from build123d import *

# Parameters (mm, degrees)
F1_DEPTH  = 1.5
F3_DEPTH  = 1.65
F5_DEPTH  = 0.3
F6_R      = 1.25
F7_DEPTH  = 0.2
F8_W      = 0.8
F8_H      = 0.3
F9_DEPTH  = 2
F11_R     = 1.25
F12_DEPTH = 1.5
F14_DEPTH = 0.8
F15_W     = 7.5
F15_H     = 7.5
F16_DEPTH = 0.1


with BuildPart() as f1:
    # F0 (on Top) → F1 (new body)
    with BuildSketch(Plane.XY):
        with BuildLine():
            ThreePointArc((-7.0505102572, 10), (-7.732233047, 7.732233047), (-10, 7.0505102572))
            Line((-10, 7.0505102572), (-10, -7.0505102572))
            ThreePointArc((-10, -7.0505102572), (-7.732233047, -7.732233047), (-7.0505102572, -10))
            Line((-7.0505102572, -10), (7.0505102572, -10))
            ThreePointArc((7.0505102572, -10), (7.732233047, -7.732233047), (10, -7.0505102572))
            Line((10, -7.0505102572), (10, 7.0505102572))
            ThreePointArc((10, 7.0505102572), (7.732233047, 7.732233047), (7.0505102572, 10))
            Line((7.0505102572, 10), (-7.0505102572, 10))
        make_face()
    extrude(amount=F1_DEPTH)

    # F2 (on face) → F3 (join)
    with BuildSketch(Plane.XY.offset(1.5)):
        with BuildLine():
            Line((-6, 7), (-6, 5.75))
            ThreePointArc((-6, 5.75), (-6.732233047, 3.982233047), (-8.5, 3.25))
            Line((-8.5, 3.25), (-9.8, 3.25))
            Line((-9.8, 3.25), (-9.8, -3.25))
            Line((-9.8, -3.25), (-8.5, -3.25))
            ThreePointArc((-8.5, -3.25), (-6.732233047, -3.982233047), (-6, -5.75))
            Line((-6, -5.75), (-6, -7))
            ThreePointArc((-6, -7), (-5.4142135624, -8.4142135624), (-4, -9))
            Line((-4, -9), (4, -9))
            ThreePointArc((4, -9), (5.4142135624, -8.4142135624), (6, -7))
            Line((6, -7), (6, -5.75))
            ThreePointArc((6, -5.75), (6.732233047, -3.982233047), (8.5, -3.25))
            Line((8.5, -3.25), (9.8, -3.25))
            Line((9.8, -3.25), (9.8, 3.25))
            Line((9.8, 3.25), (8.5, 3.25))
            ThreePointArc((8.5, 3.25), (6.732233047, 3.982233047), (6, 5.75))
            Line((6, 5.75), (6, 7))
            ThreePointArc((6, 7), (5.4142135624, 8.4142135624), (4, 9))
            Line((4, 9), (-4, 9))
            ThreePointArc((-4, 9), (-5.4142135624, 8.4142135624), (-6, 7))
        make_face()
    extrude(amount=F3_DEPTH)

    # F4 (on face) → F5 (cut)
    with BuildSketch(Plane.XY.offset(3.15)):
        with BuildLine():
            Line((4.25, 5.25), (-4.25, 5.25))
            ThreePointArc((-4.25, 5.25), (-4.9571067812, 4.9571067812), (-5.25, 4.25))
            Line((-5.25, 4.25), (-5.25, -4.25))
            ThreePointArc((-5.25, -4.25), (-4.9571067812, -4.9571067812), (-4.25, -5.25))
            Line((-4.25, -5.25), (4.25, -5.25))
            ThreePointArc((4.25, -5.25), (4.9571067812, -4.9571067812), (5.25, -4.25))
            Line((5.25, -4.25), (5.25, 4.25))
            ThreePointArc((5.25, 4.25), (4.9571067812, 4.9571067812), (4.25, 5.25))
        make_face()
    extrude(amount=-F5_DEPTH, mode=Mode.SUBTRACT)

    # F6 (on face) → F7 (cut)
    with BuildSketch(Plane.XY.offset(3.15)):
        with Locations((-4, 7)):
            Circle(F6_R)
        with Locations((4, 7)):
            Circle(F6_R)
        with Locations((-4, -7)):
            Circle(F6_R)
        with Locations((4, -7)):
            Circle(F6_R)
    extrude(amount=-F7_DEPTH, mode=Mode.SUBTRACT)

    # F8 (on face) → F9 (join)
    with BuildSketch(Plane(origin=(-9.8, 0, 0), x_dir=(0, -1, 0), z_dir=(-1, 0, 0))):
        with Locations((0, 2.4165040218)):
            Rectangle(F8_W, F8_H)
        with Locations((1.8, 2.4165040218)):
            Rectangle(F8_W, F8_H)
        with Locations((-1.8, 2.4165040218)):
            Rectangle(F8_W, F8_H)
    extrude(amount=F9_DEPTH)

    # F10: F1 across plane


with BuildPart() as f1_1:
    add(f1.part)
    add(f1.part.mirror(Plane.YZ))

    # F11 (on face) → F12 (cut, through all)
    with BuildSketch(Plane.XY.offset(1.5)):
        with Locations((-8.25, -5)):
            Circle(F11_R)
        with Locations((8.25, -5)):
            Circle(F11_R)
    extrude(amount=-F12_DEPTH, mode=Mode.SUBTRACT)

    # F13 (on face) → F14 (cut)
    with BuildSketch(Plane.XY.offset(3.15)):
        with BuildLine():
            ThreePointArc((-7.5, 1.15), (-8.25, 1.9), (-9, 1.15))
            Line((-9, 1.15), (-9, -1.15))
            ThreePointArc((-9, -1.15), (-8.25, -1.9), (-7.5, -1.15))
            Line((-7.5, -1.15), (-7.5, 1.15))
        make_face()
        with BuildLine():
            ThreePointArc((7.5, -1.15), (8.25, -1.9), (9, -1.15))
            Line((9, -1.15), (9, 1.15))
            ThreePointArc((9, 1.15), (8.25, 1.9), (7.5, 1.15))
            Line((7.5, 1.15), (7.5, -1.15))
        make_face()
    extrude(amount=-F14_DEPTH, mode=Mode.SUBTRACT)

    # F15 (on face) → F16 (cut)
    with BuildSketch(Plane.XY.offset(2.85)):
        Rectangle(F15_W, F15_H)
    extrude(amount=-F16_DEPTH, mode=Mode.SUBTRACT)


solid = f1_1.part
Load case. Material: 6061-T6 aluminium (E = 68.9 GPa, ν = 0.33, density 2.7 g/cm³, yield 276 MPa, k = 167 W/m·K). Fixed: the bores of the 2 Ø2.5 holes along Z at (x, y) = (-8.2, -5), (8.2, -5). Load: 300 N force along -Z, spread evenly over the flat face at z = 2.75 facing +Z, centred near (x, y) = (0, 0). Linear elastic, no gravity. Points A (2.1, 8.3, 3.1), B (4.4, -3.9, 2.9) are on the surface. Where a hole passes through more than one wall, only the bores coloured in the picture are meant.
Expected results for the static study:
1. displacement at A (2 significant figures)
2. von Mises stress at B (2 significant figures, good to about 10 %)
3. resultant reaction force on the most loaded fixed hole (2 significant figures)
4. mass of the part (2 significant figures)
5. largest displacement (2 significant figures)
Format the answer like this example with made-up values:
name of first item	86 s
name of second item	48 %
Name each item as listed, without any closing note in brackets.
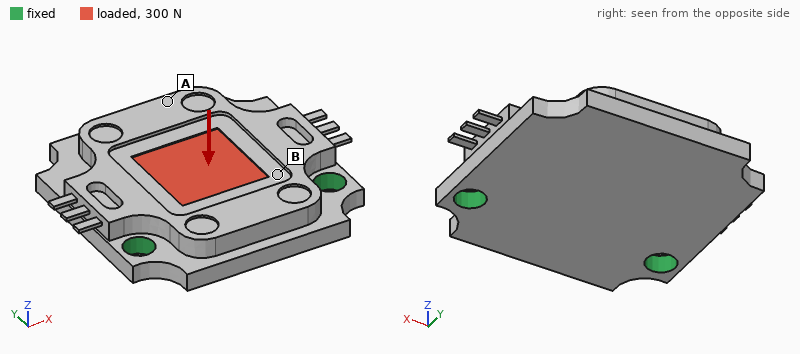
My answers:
displacement at A	75 µm
von Mises stress at B	55 MPa
resultant reaction force on the most loaded fixed hole	190 N
mass of the part	2.5 g
largest displacement	84 µm
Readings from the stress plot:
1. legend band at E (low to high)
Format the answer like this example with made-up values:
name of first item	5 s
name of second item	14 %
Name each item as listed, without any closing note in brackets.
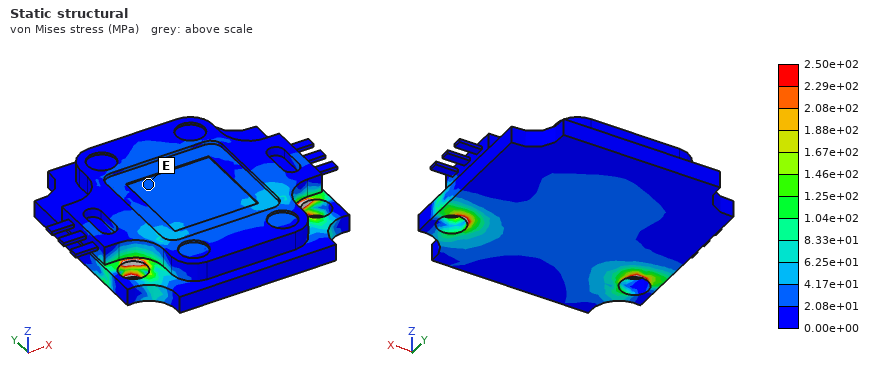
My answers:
legend band at E	2.08e+01 to 4.17e+01 MPa
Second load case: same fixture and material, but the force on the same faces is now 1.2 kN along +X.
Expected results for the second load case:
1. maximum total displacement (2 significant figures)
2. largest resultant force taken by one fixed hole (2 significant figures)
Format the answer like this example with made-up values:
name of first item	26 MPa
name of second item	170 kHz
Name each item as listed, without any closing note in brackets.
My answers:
maximum total displacement	11 µm
largest resultant force taken by one fixed hole	710 N
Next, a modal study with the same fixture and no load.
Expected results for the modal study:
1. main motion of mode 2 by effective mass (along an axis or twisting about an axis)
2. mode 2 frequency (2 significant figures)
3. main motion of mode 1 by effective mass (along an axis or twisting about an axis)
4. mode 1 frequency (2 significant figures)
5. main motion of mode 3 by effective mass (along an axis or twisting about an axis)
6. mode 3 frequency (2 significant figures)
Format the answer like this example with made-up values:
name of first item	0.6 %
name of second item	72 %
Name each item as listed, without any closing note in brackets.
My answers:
main motion of mode 2 by effective mass	twisting about Y
mode 2 frequency	23 kHz
main motion of mode 1 by effective mass	along Z
mode 1 frequency	7100 Hz
main motion of mode 3 by effective mass	along Z
mode 3 frequency	36 kHz
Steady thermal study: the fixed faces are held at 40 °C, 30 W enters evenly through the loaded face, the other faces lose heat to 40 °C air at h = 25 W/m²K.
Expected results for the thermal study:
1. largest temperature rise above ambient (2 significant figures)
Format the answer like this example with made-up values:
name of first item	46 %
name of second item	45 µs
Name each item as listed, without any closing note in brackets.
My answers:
largest temperature rise above ambient	35 K
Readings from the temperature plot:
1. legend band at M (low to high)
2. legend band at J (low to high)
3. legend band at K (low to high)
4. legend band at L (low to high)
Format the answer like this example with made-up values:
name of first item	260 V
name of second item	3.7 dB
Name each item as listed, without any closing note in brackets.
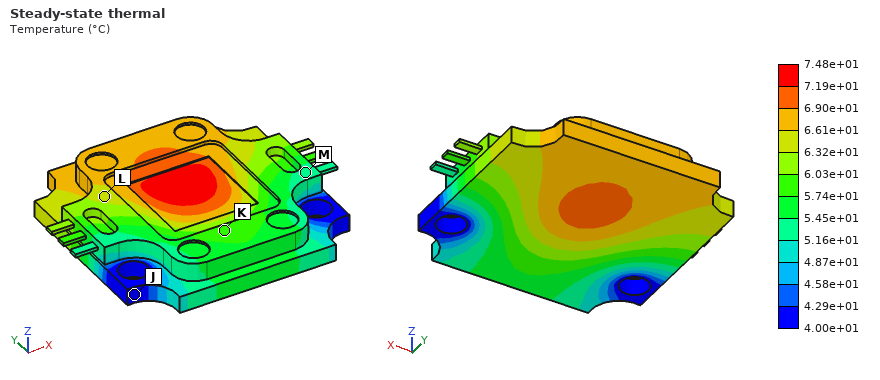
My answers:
legend band at M	5.16e+01 to 5.45e+01 °C
legend band at J	4.00e+01 to 4.29e+01 °C
legend band at K	5.74e+01 to 6.03e+01 °C
legend band at L	6.32e+01 to 6.61e+01 °C
